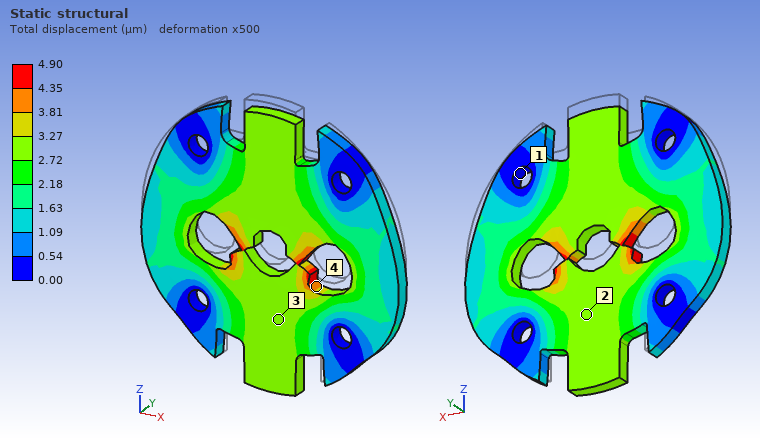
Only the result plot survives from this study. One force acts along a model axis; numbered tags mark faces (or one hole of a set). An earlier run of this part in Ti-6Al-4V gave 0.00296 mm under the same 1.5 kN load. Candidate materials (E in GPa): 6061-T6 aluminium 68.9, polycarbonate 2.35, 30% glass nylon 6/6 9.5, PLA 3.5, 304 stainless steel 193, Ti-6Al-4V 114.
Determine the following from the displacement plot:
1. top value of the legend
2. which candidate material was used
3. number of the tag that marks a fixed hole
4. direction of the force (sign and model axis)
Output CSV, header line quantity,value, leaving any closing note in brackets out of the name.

quantity,value
top value of the legend,4.90 µm
which candidate material was used,6061-T6 aluminium
number of the tag that marks a fixed hole,1
direction of the force,-Z
